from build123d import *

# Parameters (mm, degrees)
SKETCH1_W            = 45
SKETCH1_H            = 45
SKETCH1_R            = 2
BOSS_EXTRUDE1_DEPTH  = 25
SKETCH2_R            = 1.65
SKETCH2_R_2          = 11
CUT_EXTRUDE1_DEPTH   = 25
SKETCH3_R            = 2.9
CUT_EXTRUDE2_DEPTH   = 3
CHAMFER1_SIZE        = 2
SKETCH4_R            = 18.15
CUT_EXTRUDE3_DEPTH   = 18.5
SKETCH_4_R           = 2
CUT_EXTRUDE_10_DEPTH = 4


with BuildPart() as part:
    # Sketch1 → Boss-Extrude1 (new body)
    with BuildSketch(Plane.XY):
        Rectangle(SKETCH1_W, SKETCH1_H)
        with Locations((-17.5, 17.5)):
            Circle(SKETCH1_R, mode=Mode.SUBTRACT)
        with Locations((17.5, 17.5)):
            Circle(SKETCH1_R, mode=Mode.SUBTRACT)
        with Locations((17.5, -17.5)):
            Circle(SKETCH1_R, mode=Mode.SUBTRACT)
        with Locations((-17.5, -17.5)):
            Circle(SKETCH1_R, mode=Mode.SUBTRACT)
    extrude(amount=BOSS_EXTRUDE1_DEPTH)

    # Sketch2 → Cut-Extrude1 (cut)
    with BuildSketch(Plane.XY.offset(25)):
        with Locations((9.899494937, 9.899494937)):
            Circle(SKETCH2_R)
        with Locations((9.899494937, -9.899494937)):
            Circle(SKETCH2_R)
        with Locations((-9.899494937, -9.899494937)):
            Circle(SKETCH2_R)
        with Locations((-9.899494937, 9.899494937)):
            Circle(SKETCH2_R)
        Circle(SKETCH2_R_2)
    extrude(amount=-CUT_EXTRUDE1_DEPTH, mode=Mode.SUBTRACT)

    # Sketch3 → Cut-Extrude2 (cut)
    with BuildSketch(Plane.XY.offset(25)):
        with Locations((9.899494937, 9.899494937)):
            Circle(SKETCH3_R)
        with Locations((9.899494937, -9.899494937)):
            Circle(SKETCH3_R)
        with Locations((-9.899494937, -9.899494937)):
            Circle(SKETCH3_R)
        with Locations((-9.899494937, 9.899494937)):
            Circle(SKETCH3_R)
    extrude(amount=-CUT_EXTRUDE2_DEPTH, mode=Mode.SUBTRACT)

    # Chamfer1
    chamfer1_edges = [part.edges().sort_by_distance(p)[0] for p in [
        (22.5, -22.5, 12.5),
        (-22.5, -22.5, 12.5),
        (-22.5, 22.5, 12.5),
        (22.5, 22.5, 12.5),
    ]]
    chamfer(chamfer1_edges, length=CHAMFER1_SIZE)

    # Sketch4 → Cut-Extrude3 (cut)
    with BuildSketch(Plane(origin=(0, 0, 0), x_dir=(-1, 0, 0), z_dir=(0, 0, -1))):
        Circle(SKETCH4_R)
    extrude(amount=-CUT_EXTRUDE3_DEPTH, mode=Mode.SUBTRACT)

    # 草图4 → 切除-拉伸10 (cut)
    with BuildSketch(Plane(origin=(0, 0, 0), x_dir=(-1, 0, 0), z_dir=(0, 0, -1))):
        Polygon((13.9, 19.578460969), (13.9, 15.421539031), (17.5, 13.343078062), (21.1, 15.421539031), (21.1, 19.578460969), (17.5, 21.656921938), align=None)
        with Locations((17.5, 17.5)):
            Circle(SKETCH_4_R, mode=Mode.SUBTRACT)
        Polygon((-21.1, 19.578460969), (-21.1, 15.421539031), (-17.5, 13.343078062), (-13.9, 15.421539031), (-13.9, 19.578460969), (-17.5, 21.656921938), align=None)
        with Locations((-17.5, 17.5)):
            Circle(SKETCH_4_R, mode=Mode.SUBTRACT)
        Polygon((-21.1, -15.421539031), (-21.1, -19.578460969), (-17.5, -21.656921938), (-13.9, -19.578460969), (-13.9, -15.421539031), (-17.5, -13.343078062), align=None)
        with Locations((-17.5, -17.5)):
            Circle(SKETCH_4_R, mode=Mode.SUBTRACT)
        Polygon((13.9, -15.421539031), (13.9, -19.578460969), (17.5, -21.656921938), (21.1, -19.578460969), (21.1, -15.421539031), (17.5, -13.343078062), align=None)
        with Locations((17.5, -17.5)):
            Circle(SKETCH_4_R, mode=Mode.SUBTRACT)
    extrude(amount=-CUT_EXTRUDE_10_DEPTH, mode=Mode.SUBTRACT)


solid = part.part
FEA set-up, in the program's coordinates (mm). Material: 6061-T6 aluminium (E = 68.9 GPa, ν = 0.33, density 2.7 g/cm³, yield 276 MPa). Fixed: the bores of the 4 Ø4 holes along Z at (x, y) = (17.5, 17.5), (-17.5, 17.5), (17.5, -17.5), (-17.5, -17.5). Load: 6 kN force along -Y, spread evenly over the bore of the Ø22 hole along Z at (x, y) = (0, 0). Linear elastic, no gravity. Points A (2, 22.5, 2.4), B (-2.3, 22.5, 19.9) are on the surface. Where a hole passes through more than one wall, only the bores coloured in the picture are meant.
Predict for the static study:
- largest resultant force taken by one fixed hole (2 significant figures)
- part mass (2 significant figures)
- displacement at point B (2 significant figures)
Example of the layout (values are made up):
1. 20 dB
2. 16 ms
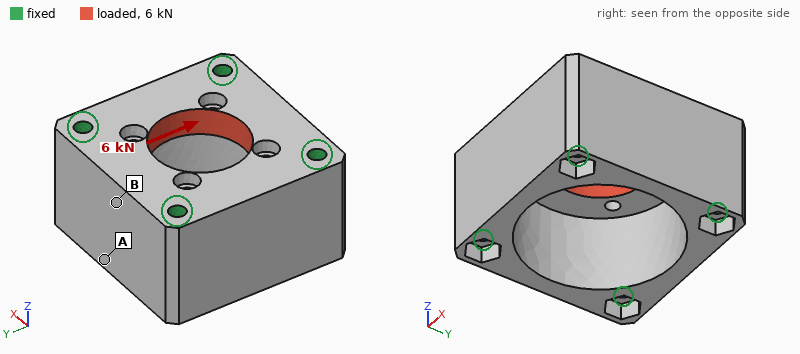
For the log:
1. 1.6 kN
2. 72 g
3. 5.6 µm
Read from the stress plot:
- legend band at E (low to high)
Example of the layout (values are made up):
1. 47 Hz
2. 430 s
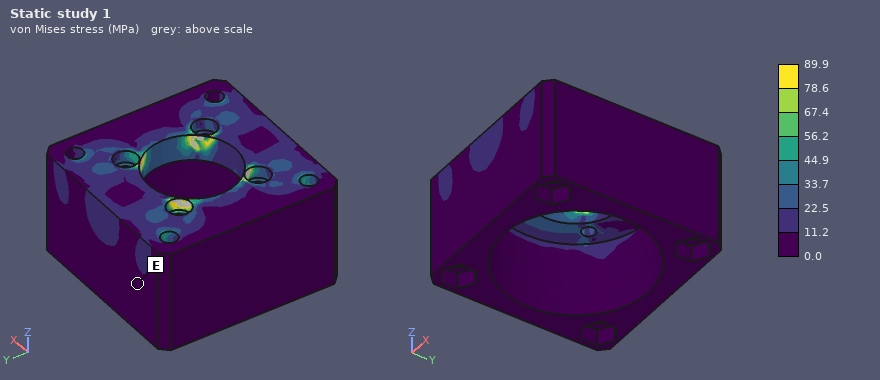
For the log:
1. 0.0 to 11.2 MPa
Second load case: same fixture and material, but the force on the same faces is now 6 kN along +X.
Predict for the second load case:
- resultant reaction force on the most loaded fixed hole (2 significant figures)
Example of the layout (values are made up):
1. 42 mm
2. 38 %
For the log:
1. 1.6 kN
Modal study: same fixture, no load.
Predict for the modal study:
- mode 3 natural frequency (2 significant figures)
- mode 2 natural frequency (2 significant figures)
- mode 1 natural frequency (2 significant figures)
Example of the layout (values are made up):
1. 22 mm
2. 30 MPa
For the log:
1. 32 kHz
2. 32 kHz
3. 25 kHz
